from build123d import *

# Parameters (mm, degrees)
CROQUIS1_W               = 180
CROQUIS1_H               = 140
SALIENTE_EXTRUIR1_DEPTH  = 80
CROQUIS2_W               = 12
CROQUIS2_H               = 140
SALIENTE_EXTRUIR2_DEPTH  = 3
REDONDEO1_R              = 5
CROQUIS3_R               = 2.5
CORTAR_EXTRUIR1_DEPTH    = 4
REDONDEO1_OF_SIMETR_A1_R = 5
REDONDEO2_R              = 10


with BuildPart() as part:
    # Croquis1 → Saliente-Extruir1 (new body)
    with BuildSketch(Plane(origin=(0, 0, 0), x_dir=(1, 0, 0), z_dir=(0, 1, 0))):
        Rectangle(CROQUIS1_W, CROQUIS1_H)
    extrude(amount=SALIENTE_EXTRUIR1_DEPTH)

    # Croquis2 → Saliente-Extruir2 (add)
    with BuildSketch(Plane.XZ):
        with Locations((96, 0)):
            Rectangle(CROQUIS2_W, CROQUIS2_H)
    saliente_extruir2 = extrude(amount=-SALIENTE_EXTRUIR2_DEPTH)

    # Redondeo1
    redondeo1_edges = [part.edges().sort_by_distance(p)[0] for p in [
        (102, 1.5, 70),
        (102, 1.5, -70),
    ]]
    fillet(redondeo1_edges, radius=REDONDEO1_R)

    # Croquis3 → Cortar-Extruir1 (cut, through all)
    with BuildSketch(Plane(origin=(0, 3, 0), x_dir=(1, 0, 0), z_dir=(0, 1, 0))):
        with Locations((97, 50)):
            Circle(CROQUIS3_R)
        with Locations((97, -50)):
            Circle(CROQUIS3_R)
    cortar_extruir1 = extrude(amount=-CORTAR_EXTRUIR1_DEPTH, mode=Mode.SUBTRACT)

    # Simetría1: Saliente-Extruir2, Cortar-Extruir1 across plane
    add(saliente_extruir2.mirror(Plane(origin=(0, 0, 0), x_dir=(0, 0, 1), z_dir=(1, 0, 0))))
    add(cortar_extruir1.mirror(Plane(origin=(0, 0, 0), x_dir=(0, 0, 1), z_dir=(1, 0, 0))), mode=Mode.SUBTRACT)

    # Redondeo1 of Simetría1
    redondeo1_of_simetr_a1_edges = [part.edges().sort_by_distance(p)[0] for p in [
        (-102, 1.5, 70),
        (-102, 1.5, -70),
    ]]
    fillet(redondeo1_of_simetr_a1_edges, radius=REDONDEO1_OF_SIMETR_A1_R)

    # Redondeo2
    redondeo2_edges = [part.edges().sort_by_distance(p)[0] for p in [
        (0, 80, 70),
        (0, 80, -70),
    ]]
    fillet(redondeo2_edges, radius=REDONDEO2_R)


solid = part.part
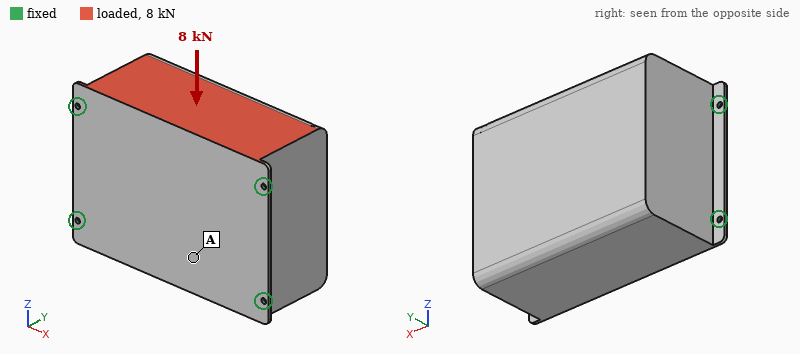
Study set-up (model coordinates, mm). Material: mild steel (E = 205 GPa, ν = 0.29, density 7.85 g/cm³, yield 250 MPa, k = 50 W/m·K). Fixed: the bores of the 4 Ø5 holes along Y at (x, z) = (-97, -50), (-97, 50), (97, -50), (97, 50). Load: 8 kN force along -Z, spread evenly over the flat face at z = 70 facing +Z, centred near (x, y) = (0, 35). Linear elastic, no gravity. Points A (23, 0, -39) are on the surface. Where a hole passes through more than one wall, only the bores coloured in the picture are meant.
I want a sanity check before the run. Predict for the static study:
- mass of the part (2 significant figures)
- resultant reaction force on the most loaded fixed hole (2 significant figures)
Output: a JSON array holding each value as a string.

["16 kg", "2.5 kN"]
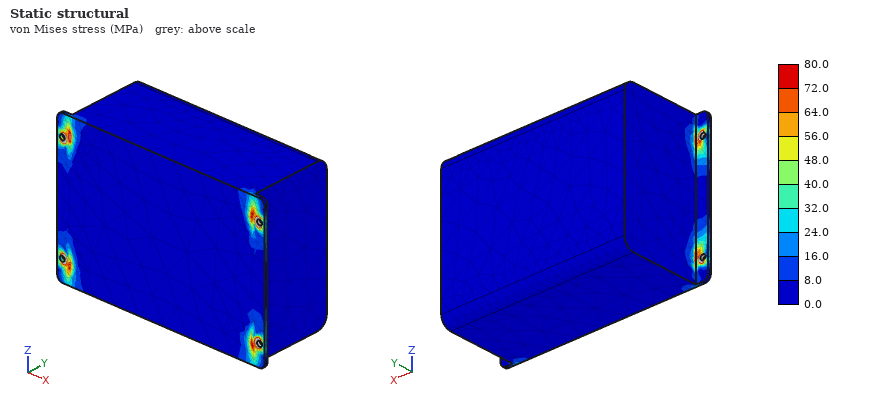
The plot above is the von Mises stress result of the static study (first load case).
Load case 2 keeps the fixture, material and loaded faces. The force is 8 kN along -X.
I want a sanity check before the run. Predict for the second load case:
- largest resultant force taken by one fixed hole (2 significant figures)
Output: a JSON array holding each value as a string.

["3.0 kN"]
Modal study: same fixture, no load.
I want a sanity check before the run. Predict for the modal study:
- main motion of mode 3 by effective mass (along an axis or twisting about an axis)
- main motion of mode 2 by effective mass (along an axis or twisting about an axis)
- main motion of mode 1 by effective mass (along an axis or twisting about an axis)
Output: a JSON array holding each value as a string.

["along X", "along Y", "along Z"]
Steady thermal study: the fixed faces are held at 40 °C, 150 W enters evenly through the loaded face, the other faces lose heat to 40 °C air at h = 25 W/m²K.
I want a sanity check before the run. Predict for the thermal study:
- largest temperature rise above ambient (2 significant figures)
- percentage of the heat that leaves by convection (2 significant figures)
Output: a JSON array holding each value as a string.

["55 K", "64 %"]
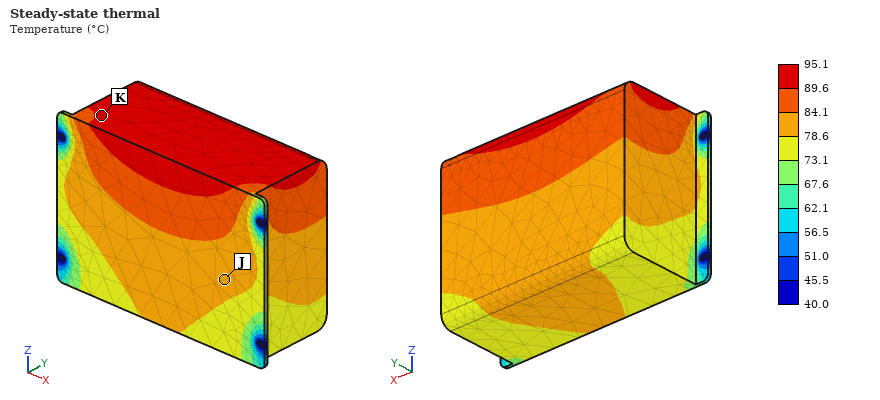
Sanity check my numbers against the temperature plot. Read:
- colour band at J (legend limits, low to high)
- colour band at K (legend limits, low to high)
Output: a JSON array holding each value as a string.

["78.6 to 84.1 °C", "89.6 to 95.1 °C"]
